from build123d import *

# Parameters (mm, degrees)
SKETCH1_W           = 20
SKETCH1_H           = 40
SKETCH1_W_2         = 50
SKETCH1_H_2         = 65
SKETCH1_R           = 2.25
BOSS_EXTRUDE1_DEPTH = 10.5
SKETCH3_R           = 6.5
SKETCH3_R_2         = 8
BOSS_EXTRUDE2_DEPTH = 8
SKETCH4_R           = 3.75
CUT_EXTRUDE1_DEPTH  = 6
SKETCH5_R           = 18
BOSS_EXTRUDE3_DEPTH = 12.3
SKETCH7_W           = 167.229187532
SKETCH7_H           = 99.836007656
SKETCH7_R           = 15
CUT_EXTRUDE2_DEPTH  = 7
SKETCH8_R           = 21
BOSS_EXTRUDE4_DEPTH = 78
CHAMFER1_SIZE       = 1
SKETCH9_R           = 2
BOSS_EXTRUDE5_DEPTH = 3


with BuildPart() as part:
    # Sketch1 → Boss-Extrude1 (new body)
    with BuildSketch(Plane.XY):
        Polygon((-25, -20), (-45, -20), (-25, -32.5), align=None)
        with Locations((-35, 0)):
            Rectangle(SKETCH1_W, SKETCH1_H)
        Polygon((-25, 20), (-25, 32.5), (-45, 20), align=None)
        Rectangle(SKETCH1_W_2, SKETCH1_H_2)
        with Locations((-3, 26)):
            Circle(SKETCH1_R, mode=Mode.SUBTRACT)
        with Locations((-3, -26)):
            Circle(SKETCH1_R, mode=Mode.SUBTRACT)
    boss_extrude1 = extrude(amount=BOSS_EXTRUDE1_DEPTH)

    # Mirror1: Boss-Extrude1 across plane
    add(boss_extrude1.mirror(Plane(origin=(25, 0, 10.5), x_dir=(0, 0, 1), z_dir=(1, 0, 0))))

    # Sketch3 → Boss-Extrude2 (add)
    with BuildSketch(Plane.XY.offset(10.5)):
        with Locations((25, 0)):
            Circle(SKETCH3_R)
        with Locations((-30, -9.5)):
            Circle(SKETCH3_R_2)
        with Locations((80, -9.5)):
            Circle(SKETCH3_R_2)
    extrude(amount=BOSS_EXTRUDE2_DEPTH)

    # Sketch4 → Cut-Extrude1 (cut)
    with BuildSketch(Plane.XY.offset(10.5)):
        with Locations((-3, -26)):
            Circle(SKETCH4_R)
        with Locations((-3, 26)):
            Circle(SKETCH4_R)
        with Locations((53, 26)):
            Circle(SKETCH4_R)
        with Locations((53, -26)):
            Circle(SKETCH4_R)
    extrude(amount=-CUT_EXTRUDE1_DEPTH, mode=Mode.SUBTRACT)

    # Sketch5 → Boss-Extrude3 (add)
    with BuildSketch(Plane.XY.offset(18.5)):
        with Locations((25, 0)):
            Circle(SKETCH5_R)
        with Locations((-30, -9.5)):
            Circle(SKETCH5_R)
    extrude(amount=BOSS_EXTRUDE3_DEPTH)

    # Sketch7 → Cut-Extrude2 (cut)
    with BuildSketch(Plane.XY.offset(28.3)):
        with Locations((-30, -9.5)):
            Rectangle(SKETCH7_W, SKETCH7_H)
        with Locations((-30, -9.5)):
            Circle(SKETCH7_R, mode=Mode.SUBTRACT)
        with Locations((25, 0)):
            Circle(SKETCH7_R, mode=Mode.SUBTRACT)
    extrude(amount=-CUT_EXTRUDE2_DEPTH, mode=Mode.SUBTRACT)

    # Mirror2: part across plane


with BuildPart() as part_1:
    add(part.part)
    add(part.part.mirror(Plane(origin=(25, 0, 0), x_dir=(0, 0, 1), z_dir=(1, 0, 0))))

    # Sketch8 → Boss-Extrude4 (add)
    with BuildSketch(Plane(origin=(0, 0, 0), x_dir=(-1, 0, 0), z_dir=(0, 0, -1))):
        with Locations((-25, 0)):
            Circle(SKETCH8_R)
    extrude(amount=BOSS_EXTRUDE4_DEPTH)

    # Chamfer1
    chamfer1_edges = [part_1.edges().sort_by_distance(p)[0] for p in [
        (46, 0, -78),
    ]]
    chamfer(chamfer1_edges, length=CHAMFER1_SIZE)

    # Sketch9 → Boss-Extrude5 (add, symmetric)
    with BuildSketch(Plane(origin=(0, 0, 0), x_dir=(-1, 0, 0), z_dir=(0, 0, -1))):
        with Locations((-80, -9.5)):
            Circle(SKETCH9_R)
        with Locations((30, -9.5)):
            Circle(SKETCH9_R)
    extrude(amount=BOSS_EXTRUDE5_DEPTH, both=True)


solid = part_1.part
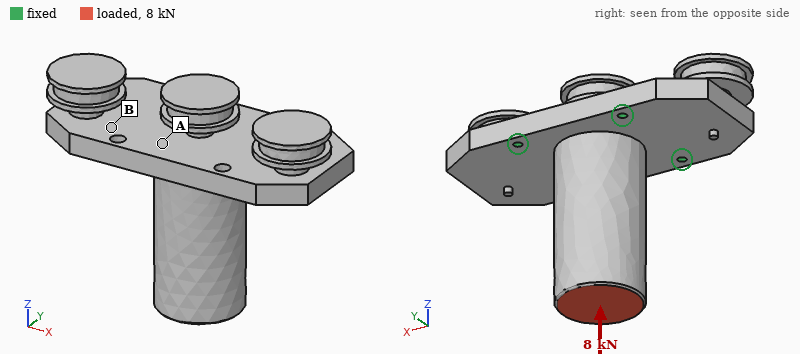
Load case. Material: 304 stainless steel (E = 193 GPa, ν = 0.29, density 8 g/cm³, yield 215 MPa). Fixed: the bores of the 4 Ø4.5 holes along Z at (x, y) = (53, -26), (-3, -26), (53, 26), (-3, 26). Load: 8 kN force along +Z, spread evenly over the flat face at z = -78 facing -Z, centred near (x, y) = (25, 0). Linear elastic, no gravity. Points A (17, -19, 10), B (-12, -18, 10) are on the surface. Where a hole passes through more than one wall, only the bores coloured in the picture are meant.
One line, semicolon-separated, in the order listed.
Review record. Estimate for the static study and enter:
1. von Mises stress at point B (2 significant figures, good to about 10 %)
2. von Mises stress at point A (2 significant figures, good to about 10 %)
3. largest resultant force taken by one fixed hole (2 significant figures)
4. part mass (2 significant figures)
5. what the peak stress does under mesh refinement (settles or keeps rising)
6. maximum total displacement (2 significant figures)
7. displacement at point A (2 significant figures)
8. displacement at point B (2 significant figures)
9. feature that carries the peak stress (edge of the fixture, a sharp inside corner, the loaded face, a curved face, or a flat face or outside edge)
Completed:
11 MPa; 26 MPa; 2.3 kN; 1.9 kg; keeps rising; 12 µm; 8.6 µm; 2.2 µm; edge of the fixture
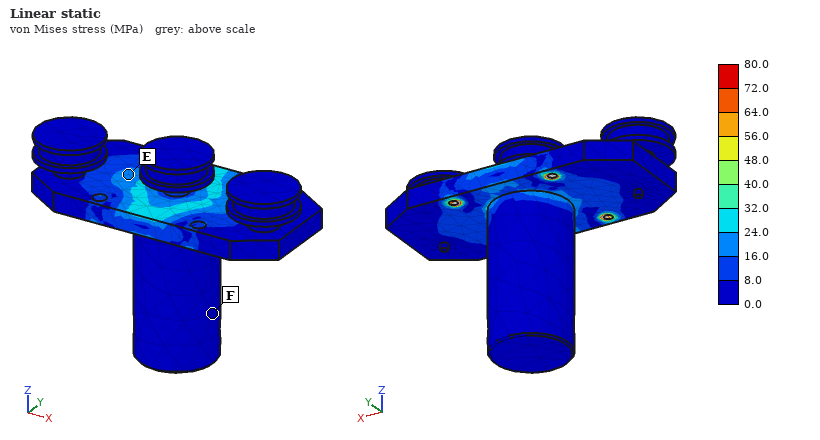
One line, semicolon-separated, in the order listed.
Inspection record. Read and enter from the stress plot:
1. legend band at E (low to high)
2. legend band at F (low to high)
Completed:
16.0 to 24.0 MPa; 0.0 to 8.0 MPa
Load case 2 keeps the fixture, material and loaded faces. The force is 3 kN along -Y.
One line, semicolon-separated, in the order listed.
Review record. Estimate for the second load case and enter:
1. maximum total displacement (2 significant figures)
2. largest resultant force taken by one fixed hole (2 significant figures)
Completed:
68 µm; 2.6 kN
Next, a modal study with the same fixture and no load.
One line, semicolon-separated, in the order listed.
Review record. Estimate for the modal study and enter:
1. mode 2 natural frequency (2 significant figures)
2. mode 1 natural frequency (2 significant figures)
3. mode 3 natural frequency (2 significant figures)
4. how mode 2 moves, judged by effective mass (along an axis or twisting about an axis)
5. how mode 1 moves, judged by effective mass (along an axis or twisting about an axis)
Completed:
2100 Hz; 1900 Hz; 2300 Hz; along X; along Y
